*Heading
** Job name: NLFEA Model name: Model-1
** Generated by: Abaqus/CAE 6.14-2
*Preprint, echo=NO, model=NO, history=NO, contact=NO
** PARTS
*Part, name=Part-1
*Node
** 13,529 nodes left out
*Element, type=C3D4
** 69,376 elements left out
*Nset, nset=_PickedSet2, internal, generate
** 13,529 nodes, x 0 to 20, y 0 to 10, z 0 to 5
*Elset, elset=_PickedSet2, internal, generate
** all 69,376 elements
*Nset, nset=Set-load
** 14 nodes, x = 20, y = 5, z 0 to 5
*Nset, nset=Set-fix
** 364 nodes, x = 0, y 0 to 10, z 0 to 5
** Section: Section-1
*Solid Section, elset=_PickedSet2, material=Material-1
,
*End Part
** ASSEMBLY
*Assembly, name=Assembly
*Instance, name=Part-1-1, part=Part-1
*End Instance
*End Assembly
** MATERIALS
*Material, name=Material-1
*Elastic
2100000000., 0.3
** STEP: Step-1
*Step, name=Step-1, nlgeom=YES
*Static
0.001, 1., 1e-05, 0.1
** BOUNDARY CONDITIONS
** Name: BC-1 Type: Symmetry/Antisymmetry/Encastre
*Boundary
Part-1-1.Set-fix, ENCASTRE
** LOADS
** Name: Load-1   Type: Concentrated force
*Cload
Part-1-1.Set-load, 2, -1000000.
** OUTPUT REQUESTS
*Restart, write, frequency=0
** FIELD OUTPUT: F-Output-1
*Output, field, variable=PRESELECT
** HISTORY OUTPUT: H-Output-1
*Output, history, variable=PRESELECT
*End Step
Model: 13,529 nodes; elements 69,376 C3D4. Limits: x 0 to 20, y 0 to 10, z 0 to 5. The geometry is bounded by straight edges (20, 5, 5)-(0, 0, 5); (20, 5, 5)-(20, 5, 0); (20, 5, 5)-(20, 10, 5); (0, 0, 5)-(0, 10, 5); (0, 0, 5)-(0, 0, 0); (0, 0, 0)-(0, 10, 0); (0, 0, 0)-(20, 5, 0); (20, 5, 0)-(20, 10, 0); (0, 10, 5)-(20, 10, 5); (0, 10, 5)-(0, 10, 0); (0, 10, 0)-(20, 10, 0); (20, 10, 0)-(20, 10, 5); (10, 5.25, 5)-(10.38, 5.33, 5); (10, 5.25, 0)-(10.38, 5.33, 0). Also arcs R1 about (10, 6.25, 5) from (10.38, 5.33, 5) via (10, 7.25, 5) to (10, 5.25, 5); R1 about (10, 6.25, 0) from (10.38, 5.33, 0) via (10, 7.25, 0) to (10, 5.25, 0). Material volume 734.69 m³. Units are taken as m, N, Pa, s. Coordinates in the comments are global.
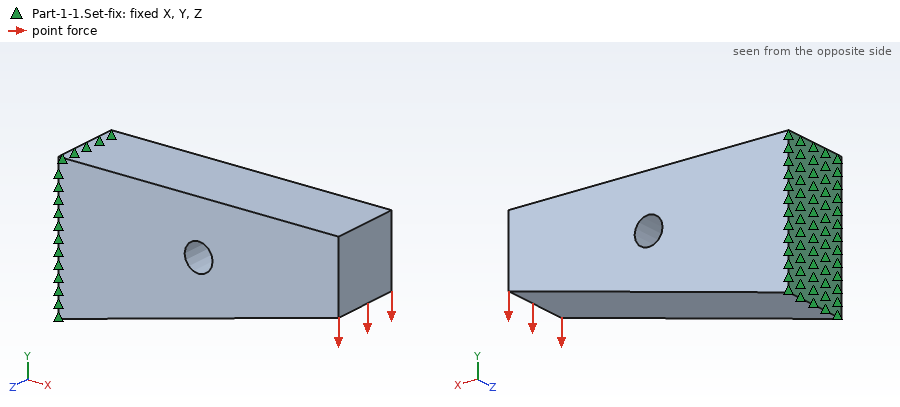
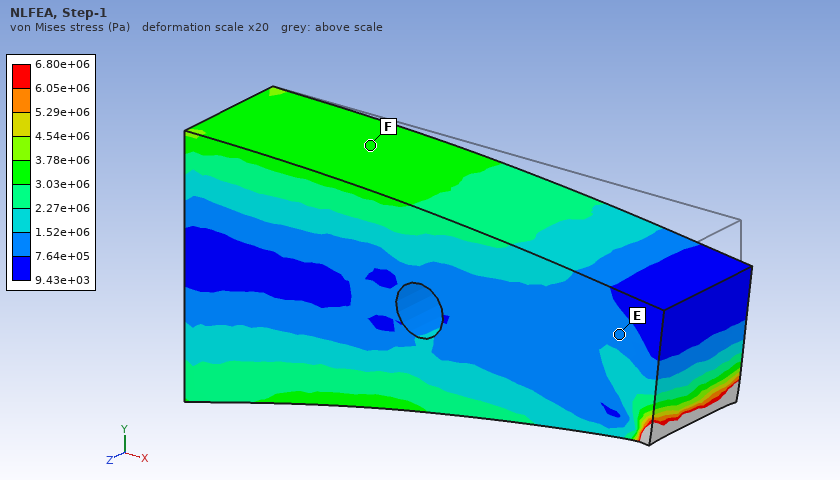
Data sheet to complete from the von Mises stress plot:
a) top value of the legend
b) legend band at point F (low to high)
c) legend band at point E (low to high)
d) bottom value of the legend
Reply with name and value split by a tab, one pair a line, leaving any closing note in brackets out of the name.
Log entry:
top value of the legend	6.80e+06 Pa
legend band at point F	3.03e+06 to 3.78e+06 Pa
legend band at point E	7.64e+05 to 1.52e+06 Pa
bottom value of the legend	9.43e+03 Pa
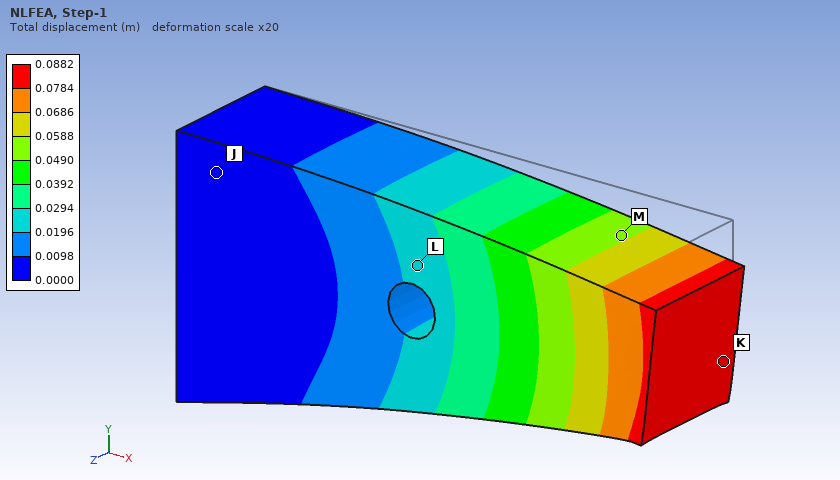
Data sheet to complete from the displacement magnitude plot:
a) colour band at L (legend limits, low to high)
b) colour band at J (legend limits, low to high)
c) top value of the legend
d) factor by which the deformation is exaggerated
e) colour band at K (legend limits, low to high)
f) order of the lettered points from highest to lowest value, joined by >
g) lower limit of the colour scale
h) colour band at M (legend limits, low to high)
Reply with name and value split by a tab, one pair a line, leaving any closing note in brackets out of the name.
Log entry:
colour band at L	0.0196 to 0.0294 m
colour band at J	0.0000 to 0.0098 m
top value of the legend	0.0882 m
factor by which the deformation is exaggerated	20
colour band at K	0.0784 to 0.0882 m
order of the lettered points from highest to lowest value, joined by >	K > M > L > J
lower limit of the colour scale	0.0000 m
colour band at M	0.0490 to 0.0588 m
